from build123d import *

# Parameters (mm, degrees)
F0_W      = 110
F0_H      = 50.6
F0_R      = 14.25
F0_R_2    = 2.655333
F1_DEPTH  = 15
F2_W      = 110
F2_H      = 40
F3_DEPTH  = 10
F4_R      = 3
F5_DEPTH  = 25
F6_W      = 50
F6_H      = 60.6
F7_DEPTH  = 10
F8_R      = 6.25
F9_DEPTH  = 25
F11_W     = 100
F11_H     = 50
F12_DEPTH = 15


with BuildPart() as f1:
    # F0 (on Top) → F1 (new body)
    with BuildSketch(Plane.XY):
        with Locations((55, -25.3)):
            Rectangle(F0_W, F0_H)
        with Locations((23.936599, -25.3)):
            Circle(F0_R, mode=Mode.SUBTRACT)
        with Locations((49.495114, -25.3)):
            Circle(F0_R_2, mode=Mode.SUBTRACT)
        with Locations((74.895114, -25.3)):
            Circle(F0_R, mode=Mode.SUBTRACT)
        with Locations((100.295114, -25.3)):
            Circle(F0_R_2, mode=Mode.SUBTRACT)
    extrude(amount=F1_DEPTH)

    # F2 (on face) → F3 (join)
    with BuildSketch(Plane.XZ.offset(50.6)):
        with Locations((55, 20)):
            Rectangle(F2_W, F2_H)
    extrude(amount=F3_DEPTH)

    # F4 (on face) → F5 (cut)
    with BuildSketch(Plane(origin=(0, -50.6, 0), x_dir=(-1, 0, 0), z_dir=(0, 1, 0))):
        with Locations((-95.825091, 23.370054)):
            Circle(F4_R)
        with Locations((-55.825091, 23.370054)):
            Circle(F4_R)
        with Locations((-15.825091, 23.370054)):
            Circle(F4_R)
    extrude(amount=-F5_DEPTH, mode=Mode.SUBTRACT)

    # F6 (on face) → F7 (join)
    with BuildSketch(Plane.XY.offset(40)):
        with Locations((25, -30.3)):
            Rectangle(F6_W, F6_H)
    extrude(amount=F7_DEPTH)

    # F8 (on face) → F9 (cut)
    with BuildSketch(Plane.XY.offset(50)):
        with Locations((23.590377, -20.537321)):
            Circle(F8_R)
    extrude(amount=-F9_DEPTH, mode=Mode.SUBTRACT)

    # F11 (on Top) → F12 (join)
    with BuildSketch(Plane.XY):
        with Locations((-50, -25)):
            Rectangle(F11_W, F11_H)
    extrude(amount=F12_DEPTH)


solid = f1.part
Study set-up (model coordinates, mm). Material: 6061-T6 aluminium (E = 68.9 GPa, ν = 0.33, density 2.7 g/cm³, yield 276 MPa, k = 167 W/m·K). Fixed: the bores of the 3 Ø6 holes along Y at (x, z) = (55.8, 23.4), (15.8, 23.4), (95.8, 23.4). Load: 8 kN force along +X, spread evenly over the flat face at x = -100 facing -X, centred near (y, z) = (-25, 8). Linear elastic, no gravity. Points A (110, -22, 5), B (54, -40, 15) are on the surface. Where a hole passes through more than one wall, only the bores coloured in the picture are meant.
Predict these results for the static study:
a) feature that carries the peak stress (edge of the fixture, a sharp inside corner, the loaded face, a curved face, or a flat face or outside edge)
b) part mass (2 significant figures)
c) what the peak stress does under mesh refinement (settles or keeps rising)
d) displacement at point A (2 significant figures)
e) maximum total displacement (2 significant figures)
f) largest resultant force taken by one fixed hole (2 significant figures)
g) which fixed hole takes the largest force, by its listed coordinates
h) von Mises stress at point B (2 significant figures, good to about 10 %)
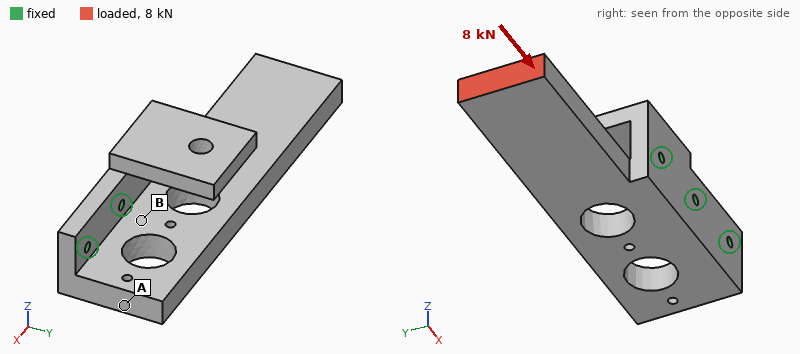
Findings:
edge of the fixture
570 g
keeps rising
0.044 mm
0.16 mm
4.6 kN
(15.8, 23.4)
13 MPa
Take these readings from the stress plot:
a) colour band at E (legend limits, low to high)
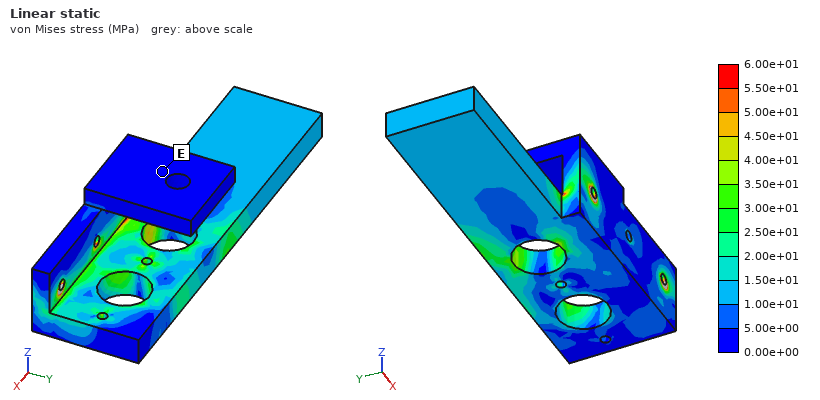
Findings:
0.00e+00 to 5.00e+00 MPa
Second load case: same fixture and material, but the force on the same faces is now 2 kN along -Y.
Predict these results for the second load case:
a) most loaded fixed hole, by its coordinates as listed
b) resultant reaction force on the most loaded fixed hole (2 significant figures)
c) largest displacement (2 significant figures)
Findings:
(15.8, 23.4)
4.8 kN
0.35 mm
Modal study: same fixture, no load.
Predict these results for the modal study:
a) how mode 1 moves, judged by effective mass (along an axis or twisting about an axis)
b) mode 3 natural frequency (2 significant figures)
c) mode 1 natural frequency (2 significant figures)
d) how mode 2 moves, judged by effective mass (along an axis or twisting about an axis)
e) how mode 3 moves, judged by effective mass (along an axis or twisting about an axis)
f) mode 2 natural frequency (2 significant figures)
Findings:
along Z
1700 Hz
620 Hz
along Y
along Z
1400 Hz
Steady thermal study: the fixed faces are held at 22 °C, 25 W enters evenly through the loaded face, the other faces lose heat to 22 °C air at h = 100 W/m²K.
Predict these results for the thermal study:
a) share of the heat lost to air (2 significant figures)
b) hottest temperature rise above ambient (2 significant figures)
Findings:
65 %
18 K
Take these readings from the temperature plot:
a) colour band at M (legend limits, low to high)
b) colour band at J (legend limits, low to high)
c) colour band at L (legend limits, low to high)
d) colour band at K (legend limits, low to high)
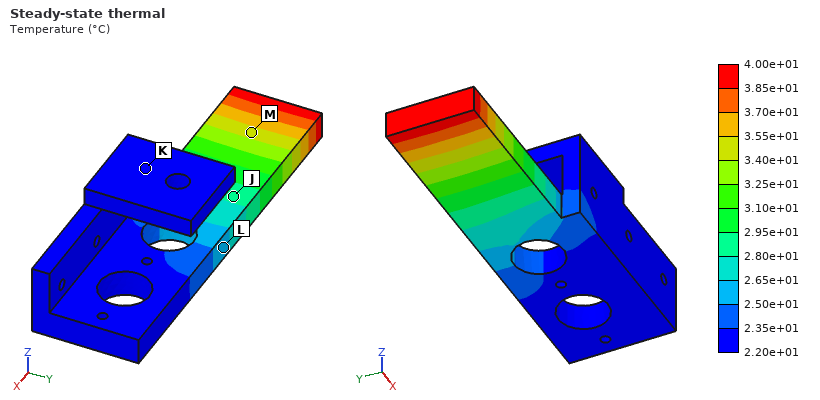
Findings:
3.40e+01 to 3.55e+01 °C
2.80e+01 to 2.95e+01 °C
2.50e+01 to 2.65e+01 °C
2.20e+01 to 2.35e+01 °C
